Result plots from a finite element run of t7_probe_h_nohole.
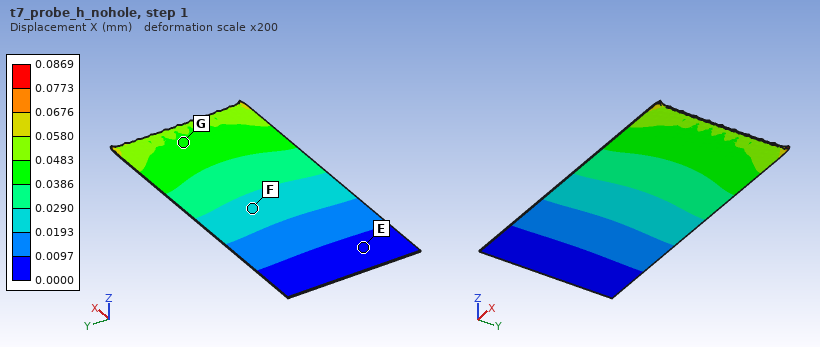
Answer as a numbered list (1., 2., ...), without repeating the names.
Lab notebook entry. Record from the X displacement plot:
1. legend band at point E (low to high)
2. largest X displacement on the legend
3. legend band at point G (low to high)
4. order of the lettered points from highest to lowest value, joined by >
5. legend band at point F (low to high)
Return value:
1. 0.0000 to 0.0097 mm
2. 0.0869 mm
3. 0.0386 to 0.0483 mm
4. G > F > E
5. 0.0193 to 0.0290 mm
